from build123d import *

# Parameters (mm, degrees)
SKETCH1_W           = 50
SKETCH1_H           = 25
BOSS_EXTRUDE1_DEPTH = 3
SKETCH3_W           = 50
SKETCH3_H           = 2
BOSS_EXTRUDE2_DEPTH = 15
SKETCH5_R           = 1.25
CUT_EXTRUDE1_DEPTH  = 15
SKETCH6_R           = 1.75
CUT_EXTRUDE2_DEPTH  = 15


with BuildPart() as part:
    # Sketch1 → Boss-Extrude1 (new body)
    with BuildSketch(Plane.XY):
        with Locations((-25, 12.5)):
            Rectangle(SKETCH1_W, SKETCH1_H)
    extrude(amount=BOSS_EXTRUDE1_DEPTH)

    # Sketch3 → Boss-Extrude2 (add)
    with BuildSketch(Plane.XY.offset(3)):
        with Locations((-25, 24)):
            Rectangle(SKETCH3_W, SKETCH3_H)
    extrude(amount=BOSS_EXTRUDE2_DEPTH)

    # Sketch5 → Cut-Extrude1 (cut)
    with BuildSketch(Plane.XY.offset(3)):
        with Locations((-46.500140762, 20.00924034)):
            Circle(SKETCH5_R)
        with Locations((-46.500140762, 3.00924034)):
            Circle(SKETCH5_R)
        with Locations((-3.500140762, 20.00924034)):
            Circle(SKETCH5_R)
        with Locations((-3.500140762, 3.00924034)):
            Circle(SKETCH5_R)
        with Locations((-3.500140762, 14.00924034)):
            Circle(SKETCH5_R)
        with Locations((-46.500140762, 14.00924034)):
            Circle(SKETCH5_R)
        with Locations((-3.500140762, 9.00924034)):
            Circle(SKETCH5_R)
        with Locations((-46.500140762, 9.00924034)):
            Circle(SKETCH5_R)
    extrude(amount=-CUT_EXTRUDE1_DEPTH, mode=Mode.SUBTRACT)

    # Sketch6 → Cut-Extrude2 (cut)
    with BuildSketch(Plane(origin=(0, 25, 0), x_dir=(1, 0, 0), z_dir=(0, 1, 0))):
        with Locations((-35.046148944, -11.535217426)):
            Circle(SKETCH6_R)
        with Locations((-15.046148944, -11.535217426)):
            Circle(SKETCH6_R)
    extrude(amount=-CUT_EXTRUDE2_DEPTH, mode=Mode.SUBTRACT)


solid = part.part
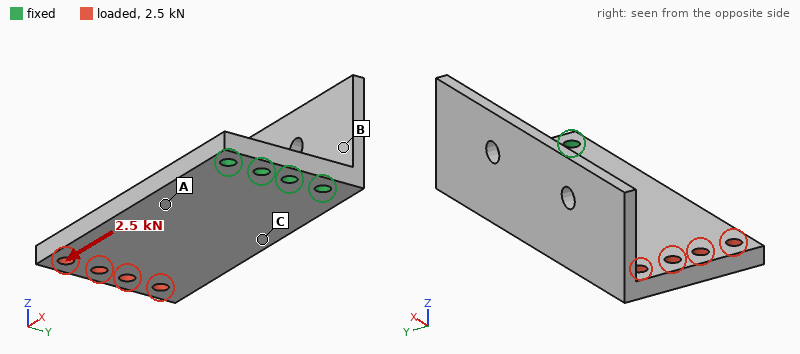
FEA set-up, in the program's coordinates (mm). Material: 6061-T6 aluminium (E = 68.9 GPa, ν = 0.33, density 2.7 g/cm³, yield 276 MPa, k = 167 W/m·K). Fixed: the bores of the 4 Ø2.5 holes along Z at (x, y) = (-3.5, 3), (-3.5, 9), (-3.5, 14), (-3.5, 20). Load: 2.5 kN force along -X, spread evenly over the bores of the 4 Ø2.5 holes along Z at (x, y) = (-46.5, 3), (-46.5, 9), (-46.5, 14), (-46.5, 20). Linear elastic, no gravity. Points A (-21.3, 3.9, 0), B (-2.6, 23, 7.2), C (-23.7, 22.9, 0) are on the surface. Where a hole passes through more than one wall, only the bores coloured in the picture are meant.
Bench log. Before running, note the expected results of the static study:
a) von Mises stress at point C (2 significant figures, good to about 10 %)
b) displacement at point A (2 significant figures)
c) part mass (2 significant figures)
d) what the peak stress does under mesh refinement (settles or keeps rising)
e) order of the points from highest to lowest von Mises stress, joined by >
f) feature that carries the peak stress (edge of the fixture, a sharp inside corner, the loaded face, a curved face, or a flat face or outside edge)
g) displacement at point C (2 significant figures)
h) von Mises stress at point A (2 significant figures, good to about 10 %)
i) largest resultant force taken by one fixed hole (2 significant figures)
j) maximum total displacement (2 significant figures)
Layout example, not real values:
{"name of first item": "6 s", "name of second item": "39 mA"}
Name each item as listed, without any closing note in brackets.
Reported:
{"von Mises stress at point C": "23 MPa", "displacement at point A": "11 µm", "part mass": "14 g", "what the peak stress does under mesh refinement": "keeps rising", "order of the points from highest to lowest von Mises stress, joined by >": "A > C > B", "feature that carries the peak stress": "edge of the fixture", "displacement at point C": "8.2 µm", "von Mises stress at point A": "42 MPa", "largest resultant force taken by one fixed hole": "740 N", "maximum total displacement": "33 µm"}
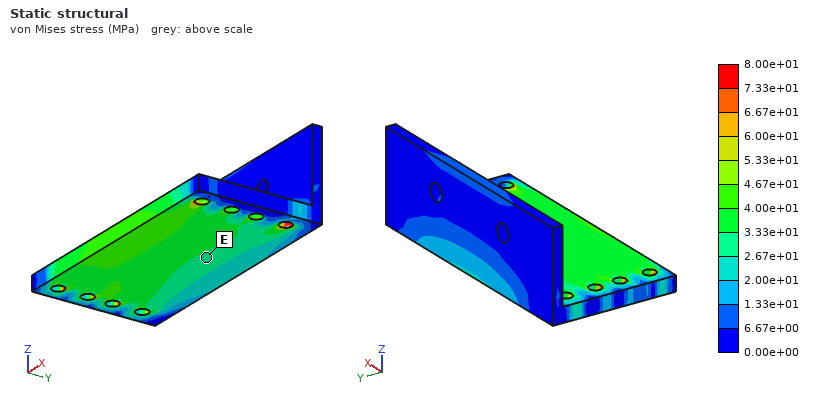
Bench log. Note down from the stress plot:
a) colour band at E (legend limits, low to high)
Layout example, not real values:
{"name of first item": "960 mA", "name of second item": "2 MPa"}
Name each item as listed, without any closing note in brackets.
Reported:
{"colour band at E": "2.67e+01 to 3.33e+01 MPa"}
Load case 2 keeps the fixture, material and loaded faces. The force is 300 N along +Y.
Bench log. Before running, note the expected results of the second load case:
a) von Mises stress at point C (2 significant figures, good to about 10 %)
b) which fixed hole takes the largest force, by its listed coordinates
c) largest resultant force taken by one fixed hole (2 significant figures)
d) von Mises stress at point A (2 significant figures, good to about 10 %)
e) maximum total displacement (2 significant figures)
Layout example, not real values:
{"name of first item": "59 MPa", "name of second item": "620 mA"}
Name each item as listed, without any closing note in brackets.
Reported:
{"von Mises stress at point C": "16 MPa", "which fixed hole takes the largest force, by its listed coordinates": "(-3.5, 20)", "largest resultant force taken by one fixed hole": "710 N", "von Mises stress at point A": "15 MPa", "maximum total displacement": "46 µm"}
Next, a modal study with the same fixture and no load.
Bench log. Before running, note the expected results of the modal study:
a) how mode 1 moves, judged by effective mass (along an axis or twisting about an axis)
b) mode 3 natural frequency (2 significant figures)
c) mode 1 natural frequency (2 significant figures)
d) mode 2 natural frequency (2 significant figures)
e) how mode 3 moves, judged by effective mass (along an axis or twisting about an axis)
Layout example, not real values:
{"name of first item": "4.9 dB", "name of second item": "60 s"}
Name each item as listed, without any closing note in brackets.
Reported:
{"how mode 1 moves, judged by effective mass": "along Z", "mode 3 natural frequency": "6100 Hz", "mode 1 natural frequency": "1600 Hz", "mode 2 natural frequency": "3000 Hz", "how mode 3 moves, judged by effective mass": "along Y"}
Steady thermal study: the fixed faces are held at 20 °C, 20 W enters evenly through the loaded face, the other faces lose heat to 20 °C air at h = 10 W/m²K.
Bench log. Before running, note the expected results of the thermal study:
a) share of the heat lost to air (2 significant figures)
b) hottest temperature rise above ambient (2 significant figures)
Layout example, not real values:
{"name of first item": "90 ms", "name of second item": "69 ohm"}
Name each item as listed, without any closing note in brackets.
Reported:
{"share of the heat lost to air": "5.8 %", "hottest temperature rise above ambient": "59 K"}
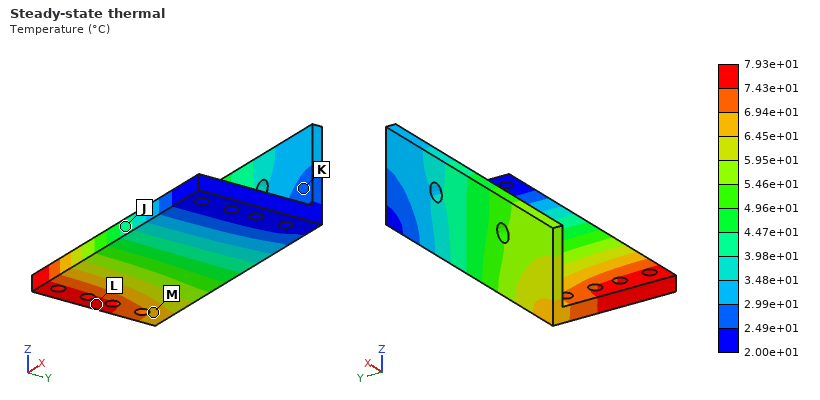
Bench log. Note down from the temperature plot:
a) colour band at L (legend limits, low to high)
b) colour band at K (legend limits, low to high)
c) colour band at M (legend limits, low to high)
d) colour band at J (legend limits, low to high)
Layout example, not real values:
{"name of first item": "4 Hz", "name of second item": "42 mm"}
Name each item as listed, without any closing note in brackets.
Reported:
{"colour band at L": "7.43e+01 to 7.93e+01 °C", "colour band at K": "2.49e+01 to 2.99e+01 °C", "colour band at M": "6.45e+01 to 6.94e+01 °C", "colour band at J": "3.98e+01 to 4.47e+01 °C"}
